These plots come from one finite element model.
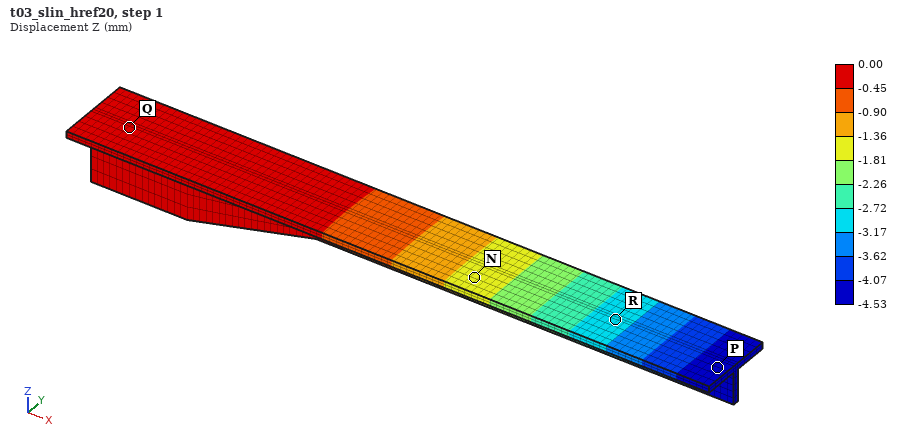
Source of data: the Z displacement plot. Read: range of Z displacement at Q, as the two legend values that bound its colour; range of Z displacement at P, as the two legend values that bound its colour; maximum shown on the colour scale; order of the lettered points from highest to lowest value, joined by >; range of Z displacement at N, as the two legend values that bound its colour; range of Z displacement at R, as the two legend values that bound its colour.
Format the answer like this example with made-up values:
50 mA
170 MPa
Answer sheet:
-0.45 to 0.00 mm
-4.53 to -4.07 mm
0.00 mm
Q > N > R > P
-1.81 to -1.36 mm
-3.17 to -2.72 mm
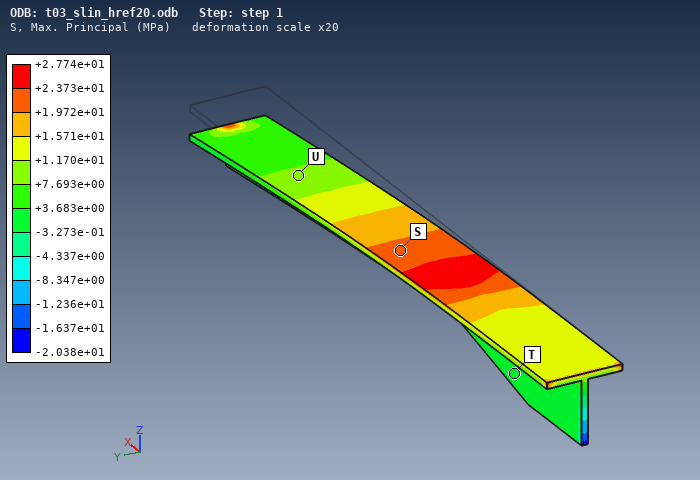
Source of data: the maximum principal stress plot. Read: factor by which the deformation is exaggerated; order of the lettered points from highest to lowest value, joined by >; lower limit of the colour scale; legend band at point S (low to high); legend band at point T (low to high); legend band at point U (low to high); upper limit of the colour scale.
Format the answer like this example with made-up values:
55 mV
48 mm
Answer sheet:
20
S > U > T
-2.038e+01 MPa
+1.972e+01 to +2.373e+01 MPa
-3.273e-01 to +3.683e+00 MPa
+7.693e+00 to +1.170e+01 MPa
+2.774e+01 MPa
